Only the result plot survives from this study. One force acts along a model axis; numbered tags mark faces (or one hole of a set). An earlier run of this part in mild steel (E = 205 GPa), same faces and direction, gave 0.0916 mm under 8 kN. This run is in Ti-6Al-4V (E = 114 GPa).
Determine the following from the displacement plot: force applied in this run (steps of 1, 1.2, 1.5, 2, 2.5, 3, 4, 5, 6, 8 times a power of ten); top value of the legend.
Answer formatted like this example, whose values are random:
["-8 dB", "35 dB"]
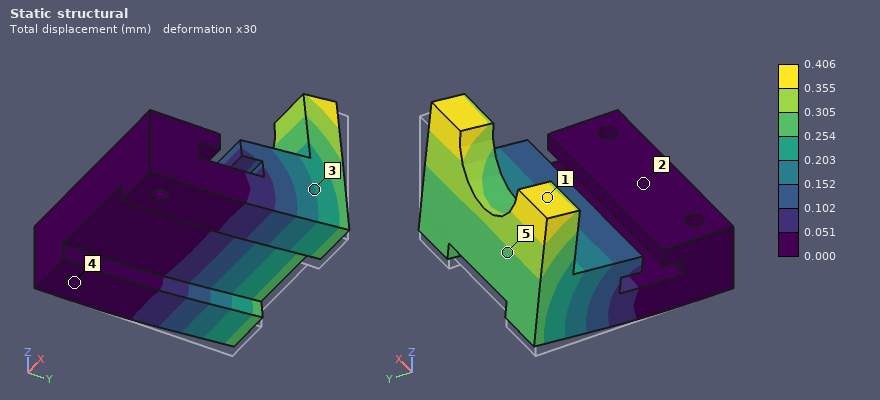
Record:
["20 kN", "0.406 mm"]
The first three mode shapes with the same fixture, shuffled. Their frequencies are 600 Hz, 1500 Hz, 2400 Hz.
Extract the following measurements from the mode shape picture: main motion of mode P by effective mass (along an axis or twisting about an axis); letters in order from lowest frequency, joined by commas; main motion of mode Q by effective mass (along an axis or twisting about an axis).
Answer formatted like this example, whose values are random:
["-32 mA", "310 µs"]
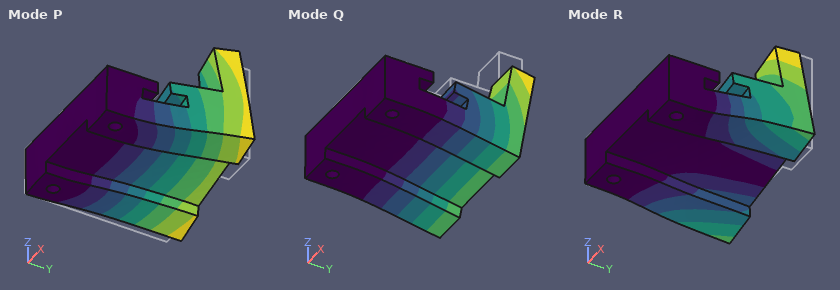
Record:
["along X", "Q, R, P", "along Z"]
